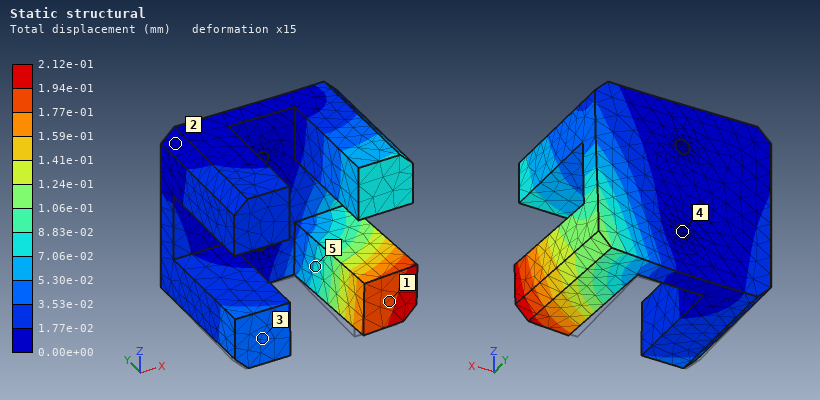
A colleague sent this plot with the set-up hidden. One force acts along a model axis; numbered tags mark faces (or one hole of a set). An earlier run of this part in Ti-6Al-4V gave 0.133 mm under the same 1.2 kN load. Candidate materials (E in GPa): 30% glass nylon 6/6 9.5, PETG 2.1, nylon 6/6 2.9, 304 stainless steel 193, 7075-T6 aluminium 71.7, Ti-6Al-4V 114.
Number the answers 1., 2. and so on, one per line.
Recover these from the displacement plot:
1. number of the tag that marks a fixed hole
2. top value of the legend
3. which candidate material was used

1. 4
2. 2.12e-01 mm
3. 7075-T6 aluminium
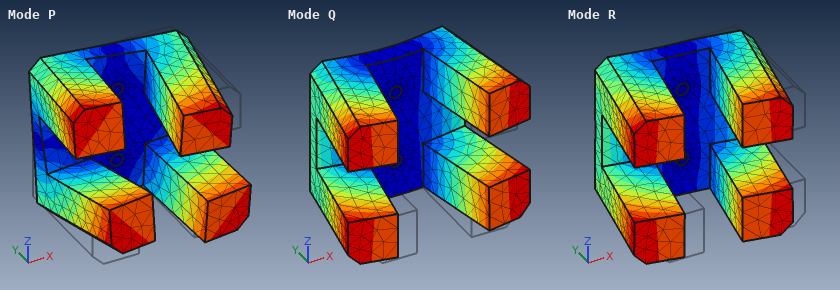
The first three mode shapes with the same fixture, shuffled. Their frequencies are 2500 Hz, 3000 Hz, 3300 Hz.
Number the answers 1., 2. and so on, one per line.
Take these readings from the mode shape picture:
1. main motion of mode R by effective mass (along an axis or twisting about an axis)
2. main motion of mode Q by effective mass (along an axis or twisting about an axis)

1. along X
2. along Y
